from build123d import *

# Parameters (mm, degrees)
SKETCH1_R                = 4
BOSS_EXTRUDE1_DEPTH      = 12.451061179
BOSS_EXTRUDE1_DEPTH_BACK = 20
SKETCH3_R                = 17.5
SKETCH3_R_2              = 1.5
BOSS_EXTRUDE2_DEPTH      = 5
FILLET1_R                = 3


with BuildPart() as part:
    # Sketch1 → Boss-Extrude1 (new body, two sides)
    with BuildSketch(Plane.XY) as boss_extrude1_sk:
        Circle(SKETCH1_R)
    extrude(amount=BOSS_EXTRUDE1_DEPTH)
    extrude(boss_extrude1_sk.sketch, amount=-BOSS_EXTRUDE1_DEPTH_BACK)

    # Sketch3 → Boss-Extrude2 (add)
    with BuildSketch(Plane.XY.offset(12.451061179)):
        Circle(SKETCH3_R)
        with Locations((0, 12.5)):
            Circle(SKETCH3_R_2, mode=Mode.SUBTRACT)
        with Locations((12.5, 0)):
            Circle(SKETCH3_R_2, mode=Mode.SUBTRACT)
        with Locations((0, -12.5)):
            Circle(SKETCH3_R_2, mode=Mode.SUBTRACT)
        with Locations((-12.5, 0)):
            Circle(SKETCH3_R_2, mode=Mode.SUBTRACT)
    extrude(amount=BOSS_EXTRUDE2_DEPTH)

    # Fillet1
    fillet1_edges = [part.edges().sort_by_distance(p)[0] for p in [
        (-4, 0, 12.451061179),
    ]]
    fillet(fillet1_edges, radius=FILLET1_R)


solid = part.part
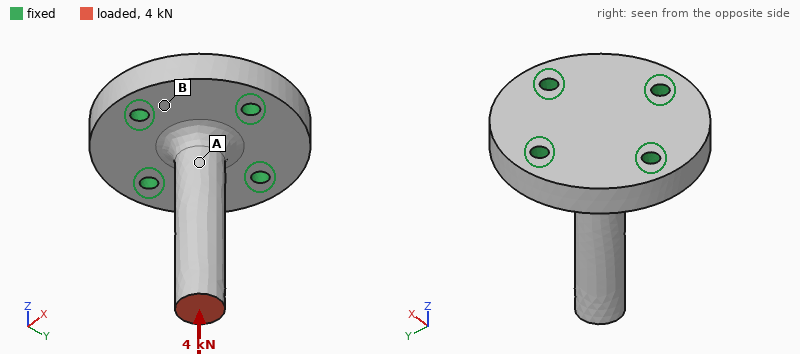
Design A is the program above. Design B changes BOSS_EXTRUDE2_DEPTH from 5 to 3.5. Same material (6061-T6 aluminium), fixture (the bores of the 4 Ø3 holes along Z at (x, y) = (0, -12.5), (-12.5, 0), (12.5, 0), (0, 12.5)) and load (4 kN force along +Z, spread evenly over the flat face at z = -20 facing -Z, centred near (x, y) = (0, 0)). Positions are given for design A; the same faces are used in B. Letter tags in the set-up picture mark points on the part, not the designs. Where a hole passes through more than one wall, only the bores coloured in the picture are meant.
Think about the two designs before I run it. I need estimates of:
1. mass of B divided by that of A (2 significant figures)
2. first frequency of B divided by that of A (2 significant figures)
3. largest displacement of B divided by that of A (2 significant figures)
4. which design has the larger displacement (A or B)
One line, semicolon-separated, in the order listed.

0.78; 0.95; 1.3; B
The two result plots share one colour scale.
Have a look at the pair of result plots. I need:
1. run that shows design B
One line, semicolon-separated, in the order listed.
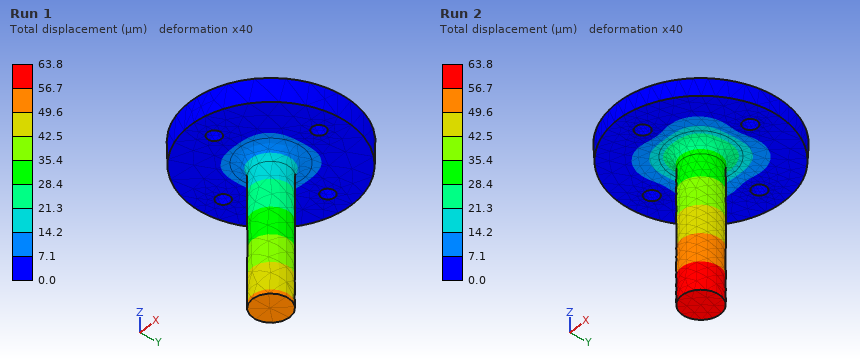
Run 2
